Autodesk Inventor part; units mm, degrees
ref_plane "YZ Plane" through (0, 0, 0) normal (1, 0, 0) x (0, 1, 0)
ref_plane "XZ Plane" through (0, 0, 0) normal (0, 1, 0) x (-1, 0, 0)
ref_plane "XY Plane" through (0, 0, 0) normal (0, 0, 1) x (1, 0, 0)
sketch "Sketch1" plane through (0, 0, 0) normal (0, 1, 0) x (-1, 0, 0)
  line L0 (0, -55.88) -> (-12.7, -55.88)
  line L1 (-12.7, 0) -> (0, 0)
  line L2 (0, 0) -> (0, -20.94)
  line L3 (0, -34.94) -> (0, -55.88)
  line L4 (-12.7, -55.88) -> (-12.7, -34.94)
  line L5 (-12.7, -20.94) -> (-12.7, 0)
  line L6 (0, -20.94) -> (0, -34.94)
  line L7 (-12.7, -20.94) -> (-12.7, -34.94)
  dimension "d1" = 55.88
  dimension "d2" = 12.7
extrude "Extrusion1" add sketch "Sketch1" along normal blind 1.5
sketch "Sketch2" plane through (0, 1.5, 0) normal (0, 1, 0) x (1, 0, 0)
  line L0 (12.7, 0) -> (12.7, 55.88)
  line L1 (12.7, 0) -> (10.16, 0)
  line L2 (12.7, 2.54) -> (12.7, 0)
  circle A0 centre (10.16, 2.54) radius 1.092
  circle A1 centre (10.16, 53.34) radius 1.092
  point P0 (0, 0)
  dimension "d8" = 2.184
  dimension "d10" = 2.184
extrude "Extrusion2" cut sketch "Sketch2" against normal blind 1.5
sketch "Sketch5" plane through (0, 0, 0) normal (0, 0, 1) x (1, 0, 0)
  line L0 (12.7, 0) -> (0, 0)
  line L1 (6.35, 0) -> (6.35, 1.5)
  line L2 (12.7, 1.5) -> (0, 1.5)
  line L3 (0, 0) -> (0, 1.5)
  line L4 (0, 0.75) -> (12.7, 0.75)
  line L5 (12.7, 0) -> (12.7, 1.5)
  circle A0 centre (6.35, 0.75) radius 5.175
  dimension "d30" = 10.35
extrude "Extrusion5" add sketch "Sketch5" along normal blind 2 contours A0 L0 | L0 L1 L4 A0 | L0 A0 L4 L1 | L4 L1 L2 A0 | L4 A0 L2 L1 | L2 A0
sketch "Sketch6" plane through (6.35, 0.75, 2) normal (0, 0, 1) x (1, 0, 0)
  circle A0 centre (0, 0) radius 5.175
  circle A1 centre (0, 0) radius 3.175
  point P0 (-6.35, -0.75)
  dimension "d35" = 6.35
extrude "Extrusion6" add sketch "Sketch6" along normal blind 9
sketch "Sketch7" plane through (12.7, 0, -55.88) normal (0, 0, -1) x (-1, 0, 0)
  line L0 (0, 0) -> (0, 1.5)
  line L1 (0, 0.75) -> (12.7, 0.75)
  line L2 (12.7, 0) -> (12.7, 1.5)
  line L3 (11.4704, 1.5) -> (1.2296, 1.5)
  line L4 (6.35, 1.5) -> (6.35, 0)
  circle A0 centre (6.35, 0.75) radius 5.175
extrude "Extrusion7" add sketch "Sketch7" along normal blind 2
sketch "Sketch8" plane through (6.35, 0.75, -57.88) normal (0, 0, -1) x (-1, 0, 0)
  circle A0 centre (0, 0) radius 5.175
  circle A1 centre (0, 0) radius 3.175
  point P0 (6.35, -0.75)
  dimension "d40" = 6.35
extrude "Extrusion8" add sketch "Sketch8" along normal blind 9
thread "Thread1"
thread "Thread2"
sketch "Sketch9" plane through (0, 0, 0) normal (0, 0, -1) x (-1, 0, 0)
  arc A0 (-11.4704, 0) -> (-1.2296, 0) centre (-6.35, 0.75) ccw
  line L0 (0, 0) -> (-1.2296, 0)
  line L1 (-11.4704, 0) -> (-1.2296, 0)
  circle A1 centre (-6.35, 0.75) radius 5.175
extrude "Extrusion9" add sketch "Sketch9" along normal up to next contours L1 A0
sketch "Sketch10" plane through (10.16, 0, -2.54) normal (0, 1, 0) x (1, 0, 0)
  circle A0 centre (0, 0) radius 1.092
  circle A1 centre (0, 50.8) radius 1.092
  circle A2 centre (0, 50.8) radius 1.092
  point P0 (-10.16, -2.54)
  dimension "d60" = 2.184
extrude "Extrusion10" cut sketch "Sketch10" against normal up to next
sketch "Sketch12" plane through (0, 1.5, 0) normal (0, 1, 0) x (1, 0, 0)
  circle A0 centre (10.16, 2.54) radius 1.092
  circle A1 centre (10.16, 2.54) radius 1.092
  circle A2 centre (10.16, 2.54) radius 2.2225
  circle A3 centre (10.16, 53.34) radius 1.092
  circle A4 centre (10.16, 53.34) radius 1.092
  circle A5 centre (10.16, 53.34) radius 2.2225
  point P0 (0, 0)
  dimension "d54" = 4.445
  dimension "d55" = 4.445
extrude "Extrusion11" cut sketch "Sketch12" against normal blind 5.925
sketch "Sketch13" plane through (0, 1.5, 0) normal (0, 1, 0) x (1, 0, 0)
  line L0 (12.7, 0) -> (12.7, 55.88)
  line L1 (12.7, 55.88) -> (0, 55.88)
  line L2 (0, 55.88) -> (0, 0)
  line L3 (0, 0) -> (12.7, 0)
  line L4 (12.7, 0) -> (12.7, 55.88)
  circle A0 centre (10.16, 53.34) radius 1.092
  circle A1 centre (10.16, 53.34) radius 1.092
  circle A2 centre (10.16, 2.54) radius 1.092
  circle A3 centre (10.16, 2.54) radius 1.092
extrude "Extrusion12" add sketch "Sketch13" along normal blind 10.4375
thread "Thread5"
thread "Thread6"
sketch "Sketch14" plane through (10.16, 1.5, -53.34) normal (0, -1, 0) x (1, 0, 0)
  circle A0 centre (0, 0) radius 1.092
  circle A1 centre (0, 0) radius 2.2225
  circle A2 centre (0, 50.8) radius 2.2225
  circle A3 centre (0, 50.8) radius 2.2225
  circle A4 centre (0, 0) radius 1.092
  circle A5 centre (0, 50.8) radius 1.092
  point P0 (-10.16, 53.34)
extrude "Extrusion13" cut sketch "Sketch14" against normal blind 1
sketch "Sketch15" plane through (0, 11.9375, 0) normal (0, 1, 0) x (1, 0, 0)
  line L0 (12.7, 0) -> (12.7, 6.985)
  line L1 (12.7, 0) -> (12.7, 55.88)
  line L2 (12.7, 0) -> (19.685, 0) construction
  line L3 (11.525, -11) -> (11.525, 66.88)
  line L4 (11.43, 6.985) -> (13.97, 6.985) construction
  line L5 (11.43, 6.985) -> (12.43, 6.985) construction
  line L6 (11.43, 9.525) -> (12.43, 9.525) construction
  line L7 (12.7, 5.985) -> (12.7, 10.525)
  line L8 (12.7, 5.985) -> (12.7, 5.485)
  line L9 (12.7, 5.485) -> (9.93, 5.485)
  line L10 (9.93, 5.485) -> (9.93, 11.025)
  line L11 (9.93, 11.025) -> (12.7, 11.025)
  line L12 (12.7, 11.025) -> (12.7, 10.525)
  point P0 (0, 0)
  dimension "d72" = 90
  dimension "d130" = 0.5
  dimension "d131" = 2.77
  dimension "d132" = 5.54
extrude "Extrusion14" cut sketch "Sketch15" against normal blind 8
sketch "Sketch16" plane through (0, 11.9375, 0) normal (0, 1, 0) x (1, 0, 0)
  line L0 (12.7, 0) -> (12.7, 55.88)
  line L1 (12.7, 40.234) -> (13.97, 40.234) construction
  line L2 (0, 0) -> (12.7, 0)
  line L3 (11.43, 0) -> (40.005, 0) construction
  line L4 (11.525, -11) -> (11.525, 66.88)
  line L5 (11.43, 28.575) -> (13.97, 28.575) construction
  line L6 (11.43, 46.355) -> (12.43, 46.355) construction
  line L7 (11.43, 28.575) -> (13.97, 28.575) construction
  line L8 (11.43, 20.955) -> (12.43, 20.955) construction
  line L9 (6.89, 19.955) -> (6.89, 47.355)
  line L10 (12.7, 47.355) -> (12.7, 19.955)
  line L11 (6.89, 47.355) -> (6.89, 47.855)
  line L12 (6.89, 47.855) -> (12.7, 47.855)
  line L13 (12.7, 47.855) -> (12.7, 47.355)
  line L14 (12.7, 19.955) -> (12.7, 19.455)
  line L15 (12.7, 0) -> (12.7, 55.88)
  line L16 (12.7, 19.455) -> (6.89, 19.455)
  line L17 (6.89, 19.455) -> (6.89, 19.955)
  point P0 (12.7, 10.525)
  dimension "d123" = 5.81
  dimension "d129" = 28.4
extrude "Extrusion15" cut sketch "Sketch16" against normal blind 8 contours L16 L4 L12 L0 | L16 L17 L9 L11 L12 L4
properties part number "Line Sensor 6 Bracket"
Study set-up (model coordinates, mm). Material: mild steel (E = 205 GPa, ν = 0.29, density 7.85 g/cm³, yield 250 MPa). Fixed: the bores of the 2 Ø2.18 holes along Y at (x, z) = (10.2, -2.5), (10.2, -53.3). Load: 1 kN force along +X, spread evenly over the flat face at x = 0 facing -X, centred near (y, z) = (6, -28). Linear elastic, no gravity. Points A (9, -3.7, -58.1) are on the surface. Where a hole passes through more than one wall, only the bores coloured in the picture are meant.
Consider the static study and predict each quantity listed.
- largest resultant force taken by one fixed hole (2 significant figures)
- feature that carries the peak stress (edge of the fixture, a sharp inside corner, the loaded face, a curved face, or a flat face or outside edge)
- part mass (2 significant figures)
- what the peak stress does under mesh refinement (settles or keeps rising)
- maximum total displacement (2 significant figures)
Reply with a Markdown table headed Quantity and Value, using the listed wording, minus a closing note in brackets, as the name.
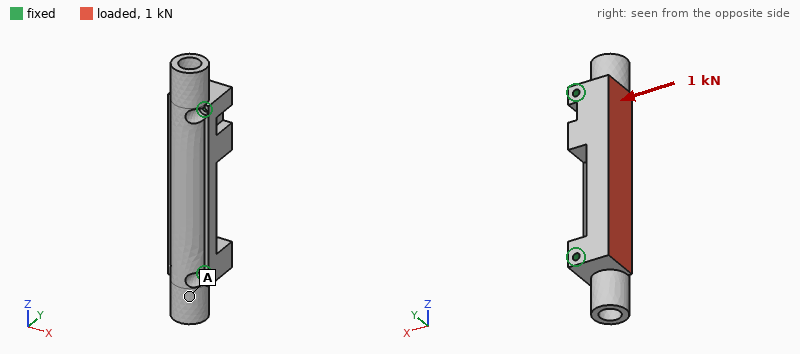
| Quantity | Value |
|---|---|
| largest resultant force taken by one fixed hole | 650 N |
| feature that carries the peak stress | edge of the fixture |
| part mass | 79 g |
| what the peak stress does under mesh refinement | keeps rising |
| maximum total displacement | 3.3 µm |
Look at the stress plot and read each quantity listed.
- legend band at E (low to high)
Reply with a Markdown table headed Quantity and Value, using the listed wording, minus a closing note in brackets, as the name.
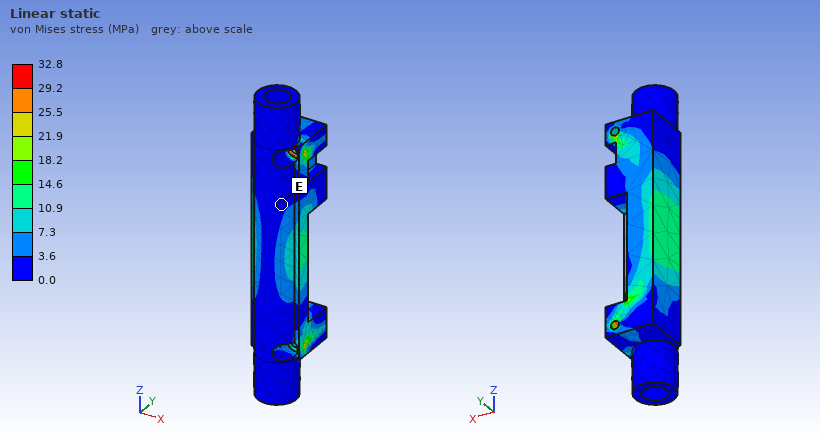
| Quantity | Value |
|---|---|
| legend band at E | 0.0 to 3.6 MPa |
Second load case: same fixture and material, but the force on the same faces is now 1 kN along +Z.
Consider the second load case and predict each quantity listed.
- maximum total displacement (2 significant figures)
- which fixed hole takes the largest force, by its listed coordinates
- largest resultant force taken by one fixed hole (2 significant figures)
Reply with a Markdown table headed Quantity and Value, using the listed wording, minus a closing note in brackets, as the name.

| Quantity | Value |
|---|---|
| maximum total displacement | 1.5 µm |
| which fixed hole takes the largest force, by its listed coordinates | (10.2, -2.5) |
| largest resultant force taken by one fixed hole | 560 N |
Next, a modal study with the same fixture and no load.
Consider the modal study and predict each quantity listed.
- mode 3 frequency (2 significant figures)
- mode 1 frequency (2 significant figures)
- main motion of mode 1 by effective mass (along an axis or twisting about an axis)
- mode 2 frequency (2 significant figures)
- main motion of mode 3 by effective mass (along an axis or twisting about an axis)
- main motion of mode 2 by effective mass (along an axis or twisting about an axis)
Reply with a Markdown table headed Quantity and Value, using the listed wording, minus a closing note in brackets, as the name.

| Quantity | Value |
|---|---|
| mode 3 frequency | 18 kHz |
| mode 1 frequency | 12 kHz |
| main motion of mode 1 by effective mass | along X |
| mode 2 frequency | 14 kHz |
| main motion of mode 3 by effective mass | twisting about Z |
| main motion of mode 2 by effective mass | along Y |
